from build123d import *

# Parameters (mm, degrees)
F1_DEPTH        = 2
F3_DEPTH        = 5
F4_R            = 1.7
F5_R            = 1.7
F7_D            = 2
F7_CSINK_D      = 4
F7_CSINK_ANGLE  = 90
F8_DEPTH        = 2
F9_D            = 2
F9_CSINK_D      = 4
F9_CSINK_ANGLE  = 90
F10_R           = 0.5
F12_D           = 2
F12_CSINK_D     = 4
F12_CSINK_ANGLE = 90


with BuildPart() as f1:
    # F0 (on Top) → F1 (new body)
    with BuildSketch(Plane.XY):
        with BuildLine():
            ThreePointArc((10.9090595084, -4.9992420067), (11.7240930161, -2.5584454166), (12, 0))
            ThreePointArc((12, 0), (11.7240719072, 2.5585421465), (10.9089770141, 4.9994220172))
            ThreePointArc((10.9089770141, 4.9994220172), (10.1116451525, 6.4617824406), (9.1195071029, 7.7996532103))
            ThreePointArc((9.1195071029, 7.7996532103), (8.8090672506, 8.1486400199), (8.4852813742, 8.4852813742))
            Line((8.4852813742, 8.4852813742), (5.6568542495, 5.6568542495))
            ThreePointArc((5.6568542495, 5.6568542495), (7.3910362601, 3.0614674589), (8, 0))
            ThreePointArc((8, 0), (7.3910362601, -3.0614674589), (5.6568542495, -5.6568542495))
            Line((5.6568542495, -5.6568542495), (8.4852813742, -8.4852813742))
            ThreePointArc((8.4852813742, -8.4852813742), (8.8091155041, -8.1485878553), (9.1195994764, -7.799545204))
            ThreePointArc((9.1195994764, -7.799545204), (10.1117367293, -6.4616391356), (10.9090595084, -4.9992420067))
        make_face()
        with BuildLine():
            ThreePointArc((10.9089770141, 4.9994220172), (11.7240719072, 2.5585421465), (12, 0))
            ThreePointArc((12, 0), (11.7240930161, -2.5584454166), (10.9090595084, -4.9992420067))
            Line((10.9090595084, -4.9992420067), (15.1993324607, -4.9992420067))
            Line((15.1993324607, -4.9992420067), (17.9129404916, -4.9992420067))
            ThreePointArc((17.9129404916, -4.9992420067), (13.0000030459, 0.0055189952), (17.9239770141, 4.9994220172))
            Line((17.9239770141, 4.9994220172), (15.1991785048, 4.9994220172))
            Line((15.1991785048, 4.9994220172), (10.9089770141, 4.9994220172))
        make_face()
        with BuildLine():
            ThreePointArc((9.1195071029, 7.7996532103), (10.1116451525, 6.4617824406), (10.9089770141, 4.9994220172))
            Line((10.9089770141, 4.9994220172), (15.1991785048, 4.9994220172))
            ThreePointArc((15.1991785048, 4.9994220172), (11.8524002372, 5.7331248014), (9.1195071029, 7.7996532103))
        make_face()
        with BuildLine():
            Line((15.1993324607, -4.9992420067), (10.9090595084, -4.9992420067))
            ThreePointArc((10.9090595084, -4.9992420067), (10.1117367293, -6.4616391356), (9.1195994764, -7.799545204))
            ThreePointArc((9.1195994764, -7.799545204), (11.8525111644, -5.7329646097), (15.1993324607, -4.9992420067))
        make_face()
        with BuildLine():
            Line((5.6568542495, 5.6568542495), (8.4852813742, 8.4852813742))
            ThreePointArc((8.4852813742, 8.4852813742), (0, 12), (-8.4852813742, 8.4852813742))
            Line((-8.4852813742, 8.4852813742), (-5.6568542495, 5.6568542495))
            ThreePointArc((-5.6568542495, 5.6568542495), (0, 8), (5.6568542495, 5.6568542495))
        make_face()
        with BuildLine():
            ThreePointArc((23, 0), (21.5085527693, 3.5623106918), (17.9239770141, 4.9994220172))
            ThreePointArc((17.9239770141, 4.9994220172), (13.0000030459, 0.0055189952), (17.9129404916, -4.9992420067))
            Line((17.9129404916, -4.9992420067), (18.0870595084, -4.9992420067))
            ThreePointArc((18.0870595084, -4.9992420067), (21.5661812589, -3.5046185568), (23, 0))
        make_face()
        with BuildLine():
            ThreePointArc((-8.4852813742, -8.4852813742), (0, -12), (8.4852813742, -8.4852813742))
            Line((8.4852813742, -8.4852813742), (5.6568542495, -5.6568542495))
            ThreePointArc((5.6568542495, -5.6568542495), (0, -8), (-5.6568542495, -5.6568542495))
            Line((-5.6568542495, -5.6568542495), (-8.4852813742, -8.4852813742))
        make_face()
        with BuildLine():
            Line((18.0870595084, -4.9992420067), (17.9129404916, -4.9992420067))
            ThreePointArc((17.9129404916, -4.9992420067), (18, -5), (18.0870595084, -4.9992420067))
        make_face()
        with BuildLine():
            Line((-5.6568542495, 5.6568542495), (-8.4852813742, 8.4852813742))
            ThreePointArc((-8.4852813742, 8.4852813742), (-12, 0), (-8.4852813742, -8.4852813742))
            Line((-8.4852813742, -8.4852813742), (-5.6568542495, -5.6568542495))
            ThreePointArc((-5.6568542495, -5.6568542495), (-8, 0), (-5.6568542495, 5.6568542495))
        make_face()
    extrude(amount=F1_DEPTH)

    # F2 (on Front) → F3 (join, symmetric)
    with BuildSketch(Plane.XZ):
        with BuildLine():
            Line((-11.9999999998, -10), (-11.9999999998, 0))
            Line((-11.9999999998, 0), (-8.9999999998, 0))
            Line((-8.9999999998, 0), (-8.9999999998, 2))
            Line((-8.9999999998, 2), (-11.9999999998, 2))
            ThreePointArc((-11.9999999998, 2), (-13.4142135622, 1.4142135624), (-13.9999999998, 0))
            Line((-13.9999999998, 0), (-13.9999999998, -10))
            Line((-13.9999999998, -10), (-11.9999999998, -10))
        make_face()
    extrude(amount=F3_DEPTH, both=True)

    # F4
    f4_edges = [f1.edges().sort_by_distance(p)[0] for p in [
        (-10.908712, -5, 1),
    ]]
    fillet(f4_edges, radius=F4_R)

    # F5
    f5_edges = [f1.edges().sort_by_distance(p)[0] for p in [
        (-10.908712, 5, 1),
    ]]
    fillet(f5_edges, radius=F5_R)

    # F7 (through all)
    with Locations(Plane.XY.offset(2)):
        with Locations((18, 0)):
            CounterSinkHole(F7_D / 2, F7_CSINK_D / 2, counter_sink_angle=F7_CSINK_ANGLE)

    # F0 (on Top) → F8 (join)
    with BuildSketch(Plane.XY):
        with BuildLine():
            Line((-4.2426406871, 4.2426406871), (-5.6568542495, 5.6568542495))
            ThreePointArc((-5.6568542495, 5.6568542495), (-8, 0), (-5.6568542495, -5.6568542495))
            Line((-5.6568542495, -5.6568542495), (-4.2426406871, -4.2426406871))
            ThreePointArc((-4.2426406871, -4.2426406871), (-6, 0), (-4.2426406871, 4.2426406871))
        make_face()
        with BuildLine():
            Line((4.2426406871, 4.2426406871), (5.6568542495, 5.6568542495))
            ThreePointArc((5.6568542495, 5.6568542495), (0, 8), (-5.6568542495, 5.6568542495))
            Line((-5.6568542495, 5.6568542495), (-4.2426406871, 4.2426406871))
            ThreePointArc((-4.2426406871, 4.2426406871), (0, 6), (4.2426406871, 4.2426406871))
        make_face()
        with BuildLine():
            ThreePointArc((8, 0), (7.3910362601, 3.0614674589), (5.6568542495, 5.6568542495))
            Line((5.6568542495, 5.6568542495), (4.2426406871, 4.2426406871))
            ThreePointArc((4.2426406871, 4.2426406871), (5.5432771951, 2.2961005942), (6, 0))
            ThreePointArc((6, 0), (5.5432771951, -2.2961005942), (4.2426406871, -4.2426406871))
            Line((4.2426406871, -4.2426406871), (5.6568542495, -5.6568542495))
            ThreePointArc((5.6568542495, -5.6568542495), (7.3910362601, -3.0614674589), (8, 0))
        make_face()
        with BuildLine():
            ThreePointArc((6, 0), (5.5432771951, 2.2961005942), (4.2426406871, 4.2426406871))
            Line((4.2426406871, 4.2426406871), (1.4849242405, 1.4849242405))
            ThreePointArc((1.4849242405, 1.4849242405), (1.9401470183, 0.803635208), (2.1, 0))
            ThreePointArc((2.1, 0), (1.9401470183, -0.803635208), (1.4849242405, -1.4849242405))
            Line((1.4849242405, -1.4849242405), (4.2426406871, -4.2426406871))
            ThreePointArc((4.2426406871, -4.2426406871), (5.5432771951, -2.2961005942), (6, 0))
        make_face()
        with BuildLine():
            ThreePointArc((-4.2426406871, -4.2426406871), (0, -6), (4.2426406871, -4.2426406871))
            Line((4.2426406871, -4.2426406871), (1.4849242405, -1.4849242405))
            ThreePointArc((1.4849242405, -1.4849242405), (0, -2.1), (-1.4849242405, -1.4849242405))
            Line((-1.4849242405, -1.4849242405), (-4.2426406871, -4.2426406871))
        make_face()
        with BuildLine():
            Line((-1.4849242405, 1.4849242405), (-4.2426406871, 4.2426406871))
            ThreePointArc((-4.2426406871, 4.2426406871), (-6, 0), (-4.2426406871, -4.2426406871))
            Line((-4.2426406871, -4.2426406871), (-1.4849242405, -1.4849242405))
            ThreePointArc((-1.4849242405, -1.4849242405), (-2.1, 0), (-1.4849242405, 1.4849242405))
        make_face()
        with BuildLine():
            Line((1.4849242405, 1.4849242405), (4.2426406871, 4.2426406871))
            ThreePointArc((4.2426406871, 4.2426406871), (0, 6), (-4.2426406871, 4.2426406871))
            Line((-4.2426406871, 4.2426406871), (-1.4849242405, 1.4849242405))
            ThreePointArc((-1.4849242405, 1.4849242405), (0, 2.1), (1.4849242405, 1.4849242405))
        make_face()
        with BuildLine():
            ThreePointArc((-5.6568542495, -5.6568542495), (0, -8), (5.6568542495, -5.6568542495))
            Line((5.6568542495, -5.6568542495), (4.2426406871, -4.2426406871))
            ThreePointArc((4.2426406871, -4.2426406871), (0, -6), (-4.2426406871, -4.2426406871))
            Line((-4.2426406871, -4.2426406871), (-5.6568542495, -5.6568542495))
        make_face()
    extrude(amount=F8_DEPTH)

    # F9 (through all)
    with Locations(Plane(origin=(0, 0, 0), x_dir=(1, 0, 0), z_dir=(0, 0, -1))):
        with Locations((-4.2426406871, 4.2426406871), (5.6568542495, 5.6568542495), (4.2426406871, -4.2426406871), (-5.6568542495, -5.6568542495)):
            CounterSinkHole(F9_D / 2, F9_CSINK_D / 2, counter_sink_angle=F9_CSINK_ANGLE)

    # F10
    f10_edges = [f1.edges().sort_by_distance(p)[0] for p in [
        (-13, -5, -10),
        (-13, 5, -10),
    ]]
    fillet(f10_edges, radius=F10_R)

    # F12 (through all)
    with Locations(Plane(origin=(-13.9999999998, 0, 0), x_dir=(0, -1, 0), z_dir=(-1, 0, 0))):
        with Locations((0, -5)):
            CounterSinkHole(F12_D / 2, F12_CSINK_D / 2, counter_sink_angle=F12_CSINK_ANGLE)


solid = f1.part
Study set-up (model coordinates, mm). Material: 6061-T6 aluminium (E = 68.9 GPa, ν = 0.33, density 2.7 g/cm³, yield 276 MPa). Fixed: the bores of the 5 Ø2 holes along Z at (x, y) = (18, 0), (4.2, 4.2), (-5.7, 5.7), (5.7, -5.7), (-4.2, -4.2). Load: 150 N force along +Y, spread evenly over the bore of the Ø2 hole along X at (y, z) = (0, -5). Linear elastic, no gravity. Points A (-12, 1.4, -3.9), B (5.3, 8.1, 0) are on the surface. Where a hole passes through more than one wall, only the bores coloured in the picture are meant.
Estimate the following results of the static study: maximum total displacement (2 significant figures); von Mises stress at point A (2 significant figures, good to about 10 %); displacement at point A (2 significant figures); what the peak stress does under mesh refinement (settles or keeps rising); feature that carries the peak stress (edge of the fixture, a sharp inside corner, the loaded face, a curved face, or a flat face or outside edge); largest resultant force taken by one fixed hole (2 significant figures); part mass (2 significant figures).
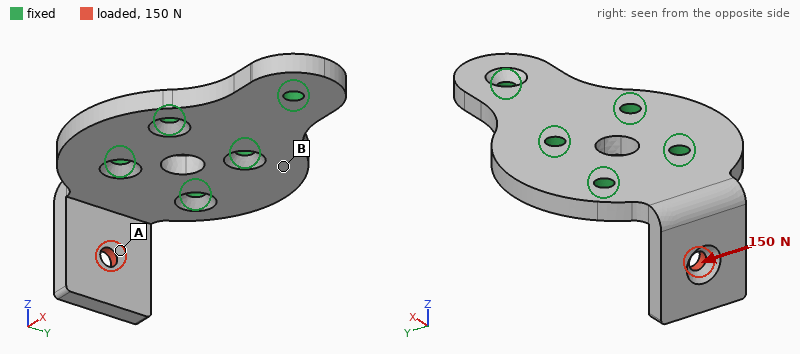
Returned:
70 µm
32 MPa
29 µm
keeps rising
edge of the fixture
160 N
3.4 g
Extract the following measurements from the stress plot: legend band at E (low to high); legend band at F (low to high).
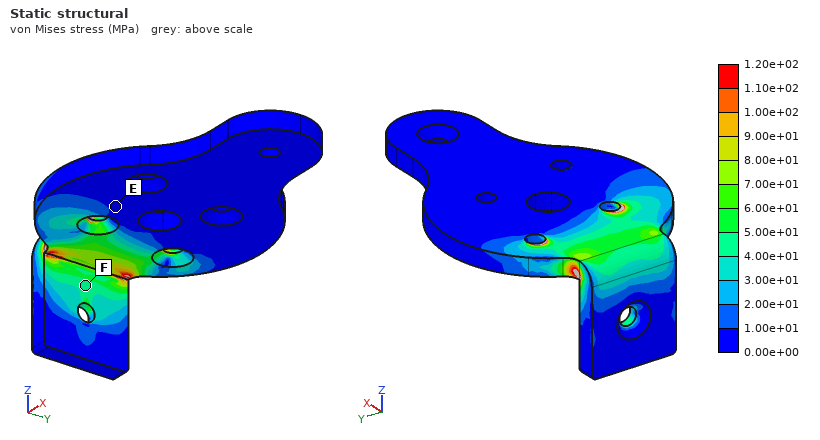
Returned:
0.00e+00 to 1.00e+01 MPa
4.00e+01 to 5.00e+01 MPa
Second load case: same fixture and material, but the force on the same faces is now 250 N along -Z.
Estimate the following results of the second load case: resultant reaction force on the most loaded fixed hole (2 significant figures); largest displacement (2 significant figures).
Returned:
210 N
0.17 mm
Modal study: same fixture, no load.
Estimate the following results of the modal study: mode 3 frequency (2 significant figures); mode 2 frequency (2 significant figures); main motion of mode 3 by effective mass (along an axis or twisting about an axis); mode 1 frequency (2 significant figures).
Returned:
17 kHz
12 kHz
along Z
6400 Hz
